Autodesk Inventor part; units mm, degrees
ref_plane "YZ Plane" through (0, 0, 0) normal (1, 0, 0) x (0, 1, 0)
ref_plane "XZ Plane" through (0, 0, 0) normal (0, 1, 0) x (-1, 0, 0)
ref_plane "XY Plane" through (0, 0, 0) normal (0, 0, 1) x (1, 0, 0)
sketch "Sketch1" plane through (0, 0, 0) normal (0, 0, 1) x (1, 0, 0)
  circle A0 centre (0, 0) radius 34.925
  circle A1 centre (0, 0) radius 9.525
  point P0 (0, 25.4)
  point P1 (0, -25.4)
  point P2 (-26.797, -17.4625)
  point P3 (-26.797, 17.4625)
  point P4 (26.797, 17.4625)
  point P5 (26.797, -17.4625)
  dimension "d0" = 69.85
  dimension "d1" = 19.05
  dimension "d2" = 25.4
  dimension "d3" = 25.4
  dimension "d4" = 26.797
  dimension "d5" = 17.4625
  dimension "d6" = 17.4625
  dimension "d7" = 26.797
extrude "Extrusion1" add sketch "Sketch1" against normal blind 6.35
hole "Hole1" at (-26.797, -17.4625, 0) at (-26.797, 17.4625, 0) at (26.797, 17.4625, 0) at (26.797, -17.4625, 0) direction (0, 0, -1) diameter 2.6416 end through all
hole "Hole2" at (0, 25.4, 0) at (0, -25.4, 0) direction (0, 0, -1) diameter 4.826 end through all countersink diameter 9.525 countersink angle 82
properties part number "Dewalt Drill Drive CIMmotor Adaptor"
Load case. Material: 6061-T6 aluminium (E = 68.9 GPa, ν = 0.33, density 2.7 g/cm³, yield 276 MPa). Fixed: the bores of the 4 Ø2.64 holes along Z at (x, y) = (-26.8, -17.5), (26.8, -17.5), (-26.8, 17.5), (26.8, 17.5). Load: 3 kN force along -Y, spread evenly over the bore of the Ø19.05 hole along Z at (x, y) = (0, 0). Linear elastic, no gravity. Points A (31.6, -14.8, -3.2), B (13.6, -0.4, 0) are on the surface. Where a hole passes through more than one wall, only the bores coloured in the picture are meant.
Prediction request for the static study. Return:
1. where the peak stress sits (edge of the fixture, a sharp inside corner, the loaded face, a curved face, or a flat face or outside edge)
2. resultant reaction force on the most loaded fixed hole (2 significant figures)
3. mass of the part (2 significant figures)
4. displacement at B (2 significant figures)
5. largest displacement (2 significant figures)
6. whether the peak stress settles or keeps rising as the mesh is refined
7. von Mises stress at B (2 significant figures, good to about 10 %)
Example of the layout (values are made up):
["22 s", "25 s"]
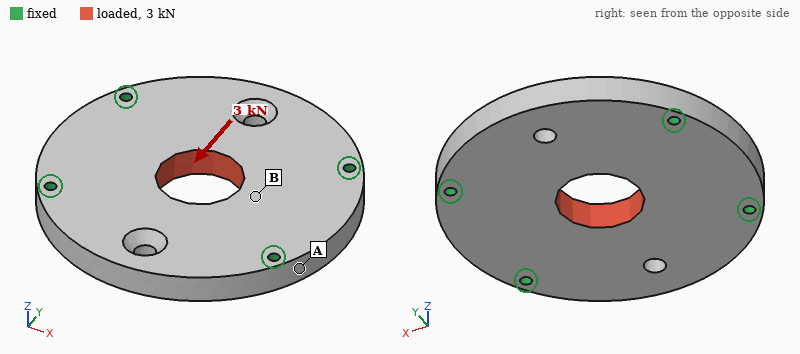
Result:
["edge of the fixture", "780 N", "59 g", "3.5 µm", "5.6 µm", "keeps rising", "12 MPa"]
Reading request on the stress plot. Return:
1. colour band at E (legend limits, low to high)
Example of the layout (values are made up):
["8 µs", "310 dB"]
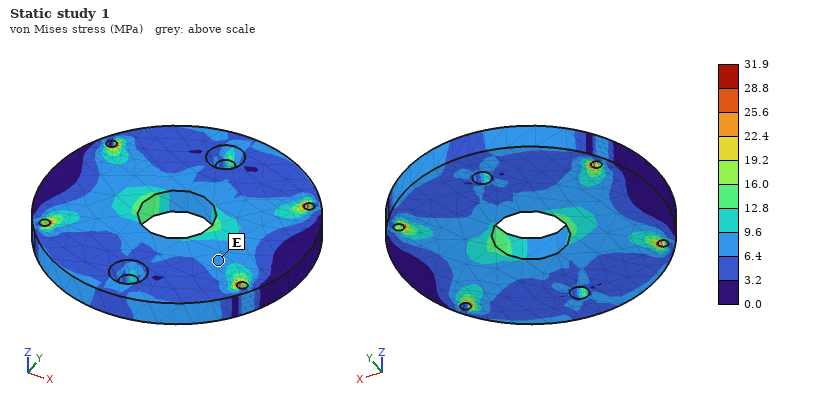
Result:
["6.4 to 9.6 MPa"]
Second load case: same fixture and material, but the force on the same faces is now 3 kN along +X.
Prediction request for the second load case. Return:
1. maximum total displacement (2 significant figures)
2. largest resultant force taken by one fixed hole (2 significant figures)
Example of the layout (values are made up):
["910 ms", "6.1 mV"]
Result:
["3.6 µm", "770 N"]
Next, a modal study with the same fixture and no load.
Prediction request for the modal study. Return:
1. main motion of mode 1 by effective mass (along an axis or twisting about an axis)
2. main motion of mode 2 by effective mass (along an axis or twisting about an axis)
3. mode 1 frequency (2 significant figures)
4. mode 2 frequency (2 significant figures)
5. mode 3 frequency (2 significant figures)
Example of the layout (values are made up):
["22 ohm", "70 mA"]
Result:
["along Z", "twisting about X", "7500 Hz", "8000 Hz", "11 kHz"]
